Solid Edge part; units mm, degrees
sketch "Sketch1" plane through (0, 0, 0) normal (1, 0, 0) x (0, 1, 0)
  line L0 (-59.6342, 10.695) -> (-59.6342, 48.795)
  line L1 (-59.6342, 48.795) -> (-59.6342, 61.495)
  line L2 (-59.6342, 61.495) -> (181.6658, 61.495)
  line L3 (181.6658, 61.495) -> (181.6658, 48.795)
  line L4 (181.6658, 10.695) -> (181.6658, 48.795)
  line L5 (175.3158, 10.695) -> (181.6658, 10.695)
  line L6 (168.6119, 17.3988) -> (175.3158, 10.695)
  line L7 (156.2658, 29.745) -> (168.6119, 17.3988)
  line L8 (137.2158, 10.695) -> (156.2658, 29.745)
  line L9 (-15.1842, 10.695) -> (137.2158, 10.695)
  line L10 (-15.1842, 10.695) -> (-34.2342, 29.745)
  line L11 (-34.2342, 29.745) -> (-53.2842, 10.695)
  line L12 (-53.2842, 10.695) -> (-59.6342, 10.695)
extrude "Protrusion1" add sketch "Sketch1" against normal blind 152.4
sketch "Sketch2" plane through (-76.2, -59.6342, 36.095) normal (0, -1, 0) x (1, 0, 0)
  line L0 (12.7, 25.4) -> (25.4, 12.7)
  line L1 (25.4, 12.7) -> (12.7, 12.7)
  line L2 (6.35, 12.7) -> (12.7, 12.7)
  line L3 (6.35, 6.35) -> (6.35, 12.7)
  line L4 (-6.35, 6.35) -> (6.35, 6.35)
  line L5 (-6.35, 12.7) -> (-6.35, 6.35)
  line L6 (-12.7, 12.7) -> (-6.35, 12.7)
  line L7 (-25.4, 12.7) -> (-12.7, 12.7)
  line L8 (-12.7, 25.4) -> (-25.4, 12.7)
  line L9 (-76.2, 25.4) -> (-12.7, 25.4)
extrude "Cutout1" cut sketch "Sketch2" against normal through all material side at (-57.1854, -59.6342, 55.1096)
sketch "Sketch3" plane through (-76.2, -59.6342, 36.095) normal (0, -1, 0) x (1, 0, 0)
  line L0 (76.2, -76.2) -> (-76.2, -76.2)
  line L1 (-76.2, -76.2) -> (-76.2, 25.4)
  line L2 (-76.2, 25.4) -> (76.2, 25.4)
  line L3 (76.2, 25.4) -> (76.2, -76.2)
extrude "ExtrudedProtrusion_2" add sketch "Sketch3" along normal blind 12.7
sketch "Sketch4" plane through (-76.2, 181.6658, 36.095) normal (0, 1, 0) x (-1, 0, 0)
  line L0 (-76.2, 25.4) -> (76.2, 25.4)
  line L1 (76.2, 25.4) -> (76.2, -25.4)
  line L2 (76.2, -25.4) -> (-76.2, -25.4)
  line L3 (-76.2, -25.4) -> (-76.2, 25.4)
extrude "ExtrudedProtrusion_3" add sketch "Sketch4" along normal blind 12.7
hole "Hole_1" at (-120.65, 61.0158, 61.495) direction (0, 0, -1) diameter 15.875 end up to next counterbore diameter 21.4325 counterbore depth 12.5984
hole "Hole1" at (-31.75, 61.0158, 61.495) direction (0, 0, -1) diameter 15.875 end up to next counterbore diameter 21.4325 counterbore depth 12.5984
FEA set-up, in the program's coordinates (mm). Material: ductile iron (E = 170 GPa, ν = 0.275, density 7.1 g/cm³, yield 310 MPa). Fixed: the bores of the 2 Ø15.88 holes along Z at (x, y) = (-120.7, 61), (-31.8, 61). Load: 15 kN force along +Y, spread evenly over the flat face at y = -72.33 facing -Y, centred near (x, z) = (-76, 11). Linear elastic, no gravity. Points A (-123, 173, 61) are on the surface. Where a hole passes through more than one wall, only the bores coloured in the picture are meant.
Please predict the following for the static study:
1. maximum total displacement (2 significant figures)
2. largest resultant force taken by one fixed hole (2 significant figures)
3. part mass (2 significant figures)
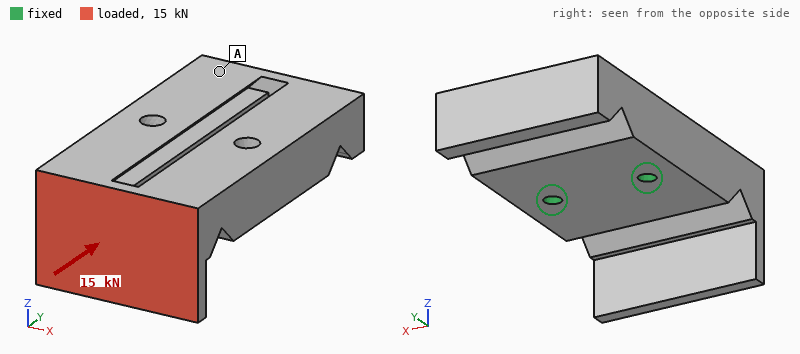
83 µm
7.6 kN
13 kg
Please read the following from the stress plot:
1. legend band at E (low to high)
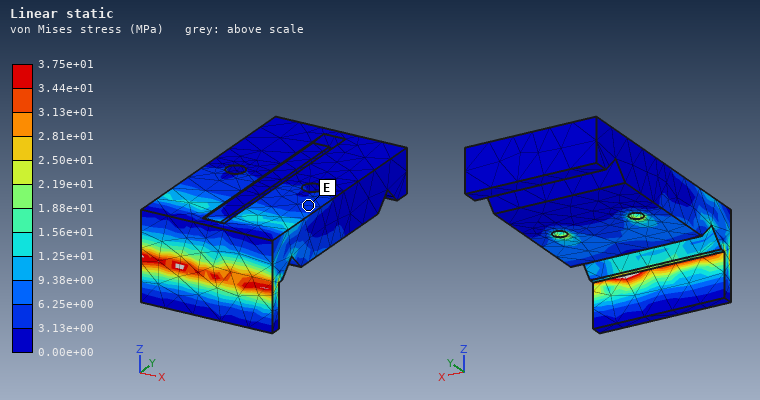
3.13e+00 to 6.25e+00 MPa
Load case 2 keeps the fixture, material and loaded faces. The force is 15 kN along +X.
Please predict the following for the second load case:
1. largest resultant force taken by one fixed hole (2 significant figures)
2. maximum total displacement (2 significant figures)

22 kN
34 µm
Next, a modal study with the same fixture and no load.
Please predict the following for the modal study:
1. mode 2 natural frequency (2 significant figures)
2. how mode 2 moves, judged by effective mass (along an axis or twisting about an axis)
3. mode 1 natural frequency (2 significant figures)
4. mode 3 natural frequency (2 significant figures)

1800 Hz
along Z
1300 Hz
2300 Hz
